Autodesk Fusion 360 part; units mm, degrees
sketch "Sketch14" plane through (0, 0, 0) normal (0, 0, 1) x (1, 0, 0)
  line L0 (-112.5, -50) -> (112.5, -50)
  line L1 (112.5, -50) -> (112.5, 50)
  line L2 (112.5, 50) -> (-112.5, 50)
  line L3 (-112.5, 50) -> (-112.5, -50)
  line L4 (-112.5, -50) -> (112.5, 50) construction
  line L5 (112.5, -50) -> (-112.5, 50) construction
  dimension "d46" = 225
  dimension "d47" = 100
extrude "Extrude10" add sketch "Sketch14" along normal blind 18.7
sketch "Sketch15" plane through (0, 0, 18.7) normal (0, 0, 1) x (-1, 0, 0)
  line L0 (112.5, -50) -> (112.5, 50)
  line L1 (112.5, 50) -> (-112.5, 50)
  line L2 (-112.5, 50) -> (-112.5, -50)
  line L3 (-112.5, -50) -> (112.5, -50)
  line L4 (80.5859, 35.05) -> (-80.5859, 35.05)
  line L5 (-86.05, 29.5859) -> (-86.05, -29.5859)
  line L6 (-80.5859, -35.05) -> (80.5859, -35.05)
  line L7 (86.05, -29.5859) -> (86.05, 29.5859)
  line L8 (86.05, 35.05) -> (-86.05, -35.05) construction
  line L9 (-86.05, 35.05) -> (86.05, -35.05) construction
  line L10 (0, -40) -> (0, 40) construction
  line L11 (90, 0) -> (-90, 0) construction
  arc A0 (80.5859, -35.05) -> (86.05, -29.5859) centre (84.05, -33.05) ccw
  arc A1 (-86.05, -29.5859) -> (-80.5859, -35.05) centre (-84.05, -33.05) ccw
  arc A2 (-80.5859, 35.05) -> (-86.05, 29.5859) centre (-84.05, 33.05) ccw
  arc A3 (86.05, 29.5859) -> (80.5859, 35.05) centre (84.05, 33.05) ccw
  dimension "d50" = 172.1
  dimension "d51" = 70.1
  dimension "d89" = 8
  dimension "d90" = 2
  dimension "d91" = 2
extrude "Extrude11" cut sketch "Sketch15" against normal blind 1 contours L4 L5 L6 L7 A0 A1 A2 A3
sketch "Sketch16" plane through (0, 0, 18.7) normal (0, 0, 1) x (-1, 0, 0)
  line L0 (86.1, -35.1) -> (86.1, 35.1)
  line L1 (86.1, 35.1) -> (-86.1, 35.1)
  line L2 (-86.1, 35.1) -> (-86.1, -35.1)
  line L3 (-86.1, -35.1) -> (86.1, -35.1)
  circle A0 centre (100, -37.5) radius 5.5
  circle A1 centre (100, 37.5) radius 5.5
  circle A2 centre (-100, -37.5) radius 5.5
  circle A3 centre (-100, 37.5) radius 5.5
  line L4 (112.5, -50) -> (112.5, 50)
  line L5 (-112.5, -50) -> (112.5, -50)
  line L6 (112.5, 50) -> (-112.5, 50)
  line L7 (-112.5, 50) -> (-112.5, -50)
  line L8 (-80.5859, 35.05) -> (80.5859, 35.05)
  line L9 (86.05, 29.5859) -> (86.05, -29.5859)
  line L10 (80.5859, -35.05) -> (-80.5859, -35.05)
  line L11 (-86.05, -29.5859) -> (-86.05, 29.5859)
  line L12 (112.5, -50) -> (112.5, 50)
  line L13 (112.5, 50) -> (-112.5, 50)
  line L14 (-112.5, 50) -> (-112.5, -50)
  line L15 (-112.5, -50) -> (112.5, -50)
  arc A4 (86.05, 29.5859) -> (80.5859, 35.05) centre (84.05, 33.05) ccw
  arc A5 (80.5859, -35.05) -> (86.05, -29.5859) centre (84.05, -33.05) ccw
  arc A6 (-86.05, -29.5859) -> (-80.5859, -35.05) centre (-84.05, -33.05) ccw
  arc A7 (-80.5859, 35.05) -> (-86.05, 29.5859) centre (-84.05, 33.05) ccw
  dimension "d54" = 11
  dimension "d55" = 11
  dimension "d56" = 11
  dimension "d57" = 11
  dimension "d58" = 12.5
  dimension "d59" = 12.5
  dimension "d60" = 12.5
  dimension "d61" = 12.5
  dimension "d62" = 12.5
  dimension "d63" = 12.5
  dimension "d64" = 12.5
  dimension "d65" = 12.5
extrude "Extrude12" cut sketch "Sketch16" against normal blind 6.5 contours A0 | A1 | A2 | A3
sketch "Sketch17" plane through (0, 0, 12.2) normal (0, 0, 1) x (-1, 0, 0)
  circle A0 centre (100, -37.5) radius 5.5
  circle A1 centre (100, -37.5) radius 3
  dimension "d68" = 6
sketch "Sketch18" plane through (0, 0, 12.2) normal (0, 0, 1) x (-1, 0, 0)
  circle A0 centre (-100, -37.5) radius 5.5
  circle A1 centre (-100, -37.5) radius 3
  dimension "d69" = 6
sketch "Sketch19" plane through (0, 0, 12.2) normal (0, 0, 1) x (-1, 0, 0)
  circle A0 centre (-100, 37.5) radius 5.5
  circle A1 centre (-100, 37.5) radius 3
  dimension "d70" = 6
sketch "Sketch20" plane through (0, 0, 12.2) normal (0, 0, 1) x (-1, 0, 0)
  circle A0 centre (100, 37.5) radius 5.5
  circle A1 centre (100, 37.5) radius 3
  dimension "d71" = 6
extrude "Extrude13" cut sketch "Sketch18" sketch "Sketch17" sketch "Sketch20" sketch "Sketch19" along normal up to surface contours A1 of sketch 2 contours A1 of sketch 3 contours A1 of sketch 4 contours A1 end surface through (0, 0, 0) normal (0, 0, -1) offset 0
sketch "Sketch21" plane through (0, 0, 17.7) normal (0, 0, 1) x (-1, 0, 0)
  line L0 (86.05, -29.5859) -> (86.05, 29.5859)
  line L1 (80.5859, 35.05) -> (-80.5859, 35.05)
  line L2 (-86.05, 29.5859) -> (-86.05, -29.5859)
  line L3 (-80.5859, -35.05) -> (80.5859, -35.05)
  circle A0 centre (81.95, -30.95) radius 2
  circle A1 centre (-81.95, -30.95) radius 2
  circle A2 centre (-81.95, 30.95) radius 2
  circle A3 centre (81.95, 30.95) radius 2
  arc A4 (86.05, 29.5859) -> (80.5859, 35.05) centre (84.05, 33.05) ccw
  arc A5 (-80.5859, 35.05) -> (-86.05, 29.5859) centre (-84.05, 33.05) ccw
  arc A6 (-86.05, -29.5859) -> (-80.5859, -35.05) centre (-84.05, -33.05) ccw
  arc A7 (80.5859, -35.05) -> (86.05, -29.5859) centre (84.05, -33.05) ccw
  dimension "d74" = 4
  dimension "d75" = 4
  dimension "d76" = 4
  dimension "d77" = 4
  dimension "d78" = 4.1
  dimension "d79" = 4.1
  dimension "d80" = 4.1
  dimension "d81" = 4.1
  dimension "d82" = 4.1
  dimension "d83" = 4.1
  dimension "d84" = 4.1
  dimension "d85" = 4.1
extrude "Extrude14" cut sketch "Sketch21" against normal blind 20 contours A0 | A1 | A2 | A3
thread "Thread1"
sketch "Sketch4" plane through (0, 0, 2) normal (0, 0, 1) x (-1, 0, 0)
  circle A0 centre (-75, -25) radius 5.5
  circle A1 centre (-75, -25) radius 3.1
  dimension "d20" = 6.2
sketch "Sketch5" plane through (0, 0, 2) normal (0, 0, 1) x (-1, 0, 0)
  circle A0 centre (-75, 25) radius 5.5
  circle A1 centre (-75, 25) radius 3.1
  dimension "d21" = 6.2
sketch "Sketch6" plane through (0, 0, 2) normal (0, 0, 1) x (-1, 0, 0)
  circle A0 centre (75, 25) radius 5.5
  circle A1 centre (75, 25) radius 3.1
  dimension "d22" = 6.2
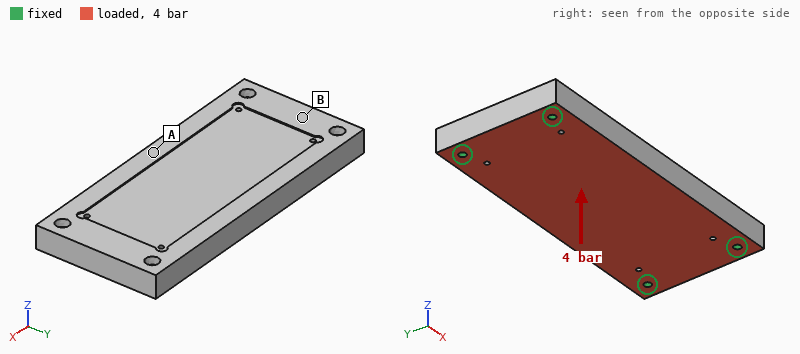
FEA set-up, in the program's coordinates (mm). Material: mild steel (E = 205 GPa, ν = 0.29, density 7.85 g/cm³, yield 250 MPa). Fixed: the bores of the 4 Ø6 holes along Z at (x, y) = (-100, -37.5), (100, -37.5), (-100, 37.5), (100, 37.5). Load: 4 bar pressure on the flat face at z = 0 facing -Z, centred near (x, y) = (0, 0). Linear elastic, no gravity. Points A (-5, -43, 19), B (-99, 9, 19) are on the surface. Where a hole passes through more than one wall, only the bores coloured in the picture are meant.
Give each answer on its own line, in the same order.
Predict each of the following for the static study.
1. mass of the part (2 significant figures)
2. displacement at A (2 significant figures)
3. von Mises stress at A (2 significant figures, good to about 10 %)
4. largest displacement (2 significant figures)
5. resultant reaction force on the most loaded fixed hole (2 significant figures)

3.2 kg
33 µm
20 MPa
33 µm
2.5 kN
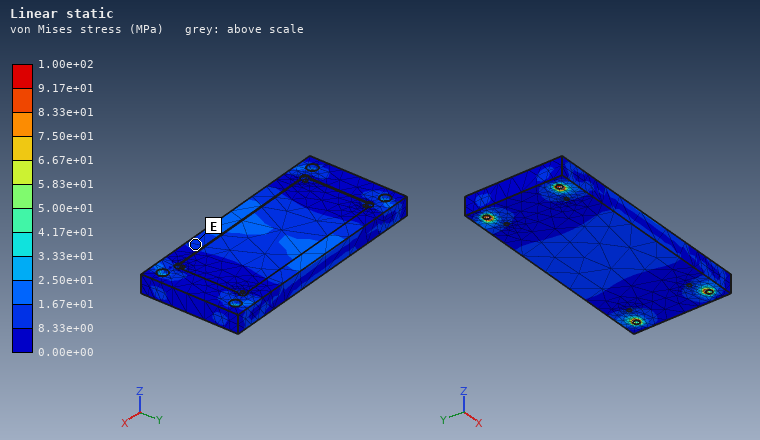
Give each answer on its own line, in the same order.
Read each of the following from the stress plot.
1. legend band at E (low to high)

8.33e+00 to 1.67e+01 MPa
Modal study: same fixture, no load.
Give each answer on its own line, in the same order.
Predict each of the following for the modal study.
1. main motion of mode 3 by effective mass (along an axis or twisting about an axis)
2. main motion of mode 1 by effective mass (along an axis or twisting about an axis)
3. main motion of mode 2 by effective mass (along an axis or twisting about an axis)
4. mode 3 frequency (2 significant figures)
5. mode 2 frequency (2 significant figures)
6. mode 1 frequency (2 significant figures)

twisting about Y
along Z
twisting about X
4700 Hz
3200 Hz
1700 Hz
